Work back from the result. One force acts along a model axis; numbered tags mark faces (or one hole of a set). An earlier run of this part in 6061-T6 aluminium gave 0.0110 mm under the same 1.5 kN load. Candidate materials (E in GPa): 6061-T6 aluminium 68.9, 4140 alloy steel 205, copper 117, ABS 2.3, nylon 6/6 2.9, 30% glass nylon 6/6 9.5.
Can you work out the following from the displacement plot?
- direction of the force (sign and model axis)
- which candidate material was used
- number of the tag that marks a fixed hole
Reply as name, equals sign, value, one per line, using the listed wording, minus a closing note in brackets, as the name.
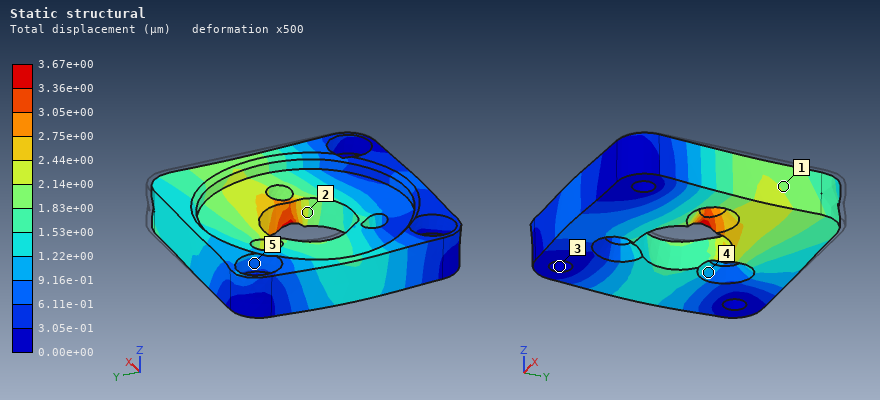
direction of the force = -X
which candidate material was used = 4140 alloy steel
number of the tag that marks a fixed hole = 3
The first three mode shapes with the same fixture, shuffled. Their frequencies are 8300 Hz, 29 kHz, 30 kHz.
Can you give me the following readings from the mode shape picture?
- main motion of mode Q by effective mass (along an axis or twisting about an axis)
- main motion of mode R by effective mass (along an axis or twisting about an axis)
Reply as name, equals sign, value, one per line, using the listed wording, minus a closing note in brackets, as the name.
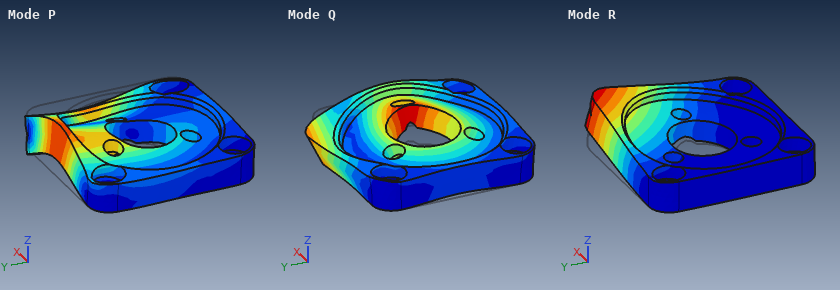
main motion of mode Q by effective mass = along Z
main motion of mode R by effective mass = along Z
